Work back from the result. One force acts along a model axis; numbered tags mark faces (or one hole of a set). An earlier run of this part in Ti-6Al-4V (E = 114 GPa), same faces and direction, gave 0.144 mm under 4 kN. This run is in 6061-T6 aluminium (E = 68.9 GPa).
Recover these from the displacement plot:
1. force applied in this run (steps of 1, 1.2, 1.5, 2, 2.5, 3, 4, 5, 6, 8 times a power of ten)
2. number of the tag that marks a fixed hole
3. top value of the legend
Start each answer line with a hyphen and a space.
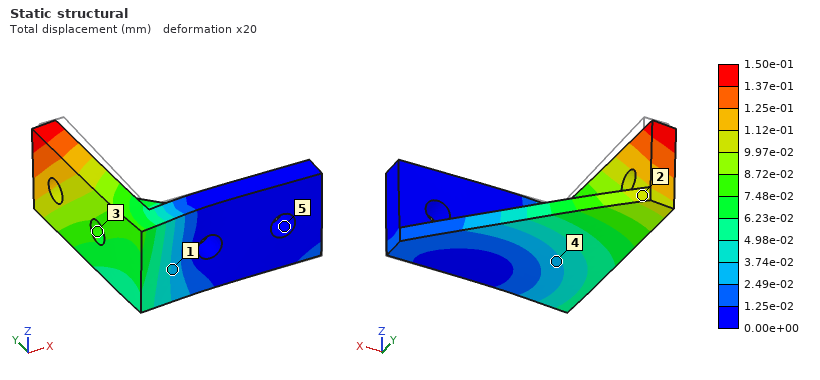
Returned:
- 2.5 kN
- 5
- 1.50e-01 mm
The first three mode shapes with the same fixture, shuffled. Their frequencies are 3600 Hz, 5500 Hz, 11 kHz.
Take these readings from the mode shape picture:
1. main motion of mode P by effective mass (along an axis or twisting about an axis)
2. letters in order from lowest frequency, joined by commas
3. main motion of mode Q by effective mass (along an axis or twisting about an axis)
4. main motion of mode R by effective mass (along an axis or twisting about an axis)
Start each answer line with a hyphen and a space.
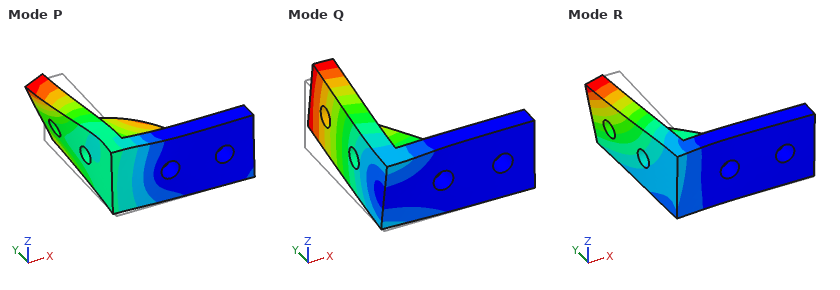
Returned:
- along Y
- Q, R, P
- along Z
- along X
